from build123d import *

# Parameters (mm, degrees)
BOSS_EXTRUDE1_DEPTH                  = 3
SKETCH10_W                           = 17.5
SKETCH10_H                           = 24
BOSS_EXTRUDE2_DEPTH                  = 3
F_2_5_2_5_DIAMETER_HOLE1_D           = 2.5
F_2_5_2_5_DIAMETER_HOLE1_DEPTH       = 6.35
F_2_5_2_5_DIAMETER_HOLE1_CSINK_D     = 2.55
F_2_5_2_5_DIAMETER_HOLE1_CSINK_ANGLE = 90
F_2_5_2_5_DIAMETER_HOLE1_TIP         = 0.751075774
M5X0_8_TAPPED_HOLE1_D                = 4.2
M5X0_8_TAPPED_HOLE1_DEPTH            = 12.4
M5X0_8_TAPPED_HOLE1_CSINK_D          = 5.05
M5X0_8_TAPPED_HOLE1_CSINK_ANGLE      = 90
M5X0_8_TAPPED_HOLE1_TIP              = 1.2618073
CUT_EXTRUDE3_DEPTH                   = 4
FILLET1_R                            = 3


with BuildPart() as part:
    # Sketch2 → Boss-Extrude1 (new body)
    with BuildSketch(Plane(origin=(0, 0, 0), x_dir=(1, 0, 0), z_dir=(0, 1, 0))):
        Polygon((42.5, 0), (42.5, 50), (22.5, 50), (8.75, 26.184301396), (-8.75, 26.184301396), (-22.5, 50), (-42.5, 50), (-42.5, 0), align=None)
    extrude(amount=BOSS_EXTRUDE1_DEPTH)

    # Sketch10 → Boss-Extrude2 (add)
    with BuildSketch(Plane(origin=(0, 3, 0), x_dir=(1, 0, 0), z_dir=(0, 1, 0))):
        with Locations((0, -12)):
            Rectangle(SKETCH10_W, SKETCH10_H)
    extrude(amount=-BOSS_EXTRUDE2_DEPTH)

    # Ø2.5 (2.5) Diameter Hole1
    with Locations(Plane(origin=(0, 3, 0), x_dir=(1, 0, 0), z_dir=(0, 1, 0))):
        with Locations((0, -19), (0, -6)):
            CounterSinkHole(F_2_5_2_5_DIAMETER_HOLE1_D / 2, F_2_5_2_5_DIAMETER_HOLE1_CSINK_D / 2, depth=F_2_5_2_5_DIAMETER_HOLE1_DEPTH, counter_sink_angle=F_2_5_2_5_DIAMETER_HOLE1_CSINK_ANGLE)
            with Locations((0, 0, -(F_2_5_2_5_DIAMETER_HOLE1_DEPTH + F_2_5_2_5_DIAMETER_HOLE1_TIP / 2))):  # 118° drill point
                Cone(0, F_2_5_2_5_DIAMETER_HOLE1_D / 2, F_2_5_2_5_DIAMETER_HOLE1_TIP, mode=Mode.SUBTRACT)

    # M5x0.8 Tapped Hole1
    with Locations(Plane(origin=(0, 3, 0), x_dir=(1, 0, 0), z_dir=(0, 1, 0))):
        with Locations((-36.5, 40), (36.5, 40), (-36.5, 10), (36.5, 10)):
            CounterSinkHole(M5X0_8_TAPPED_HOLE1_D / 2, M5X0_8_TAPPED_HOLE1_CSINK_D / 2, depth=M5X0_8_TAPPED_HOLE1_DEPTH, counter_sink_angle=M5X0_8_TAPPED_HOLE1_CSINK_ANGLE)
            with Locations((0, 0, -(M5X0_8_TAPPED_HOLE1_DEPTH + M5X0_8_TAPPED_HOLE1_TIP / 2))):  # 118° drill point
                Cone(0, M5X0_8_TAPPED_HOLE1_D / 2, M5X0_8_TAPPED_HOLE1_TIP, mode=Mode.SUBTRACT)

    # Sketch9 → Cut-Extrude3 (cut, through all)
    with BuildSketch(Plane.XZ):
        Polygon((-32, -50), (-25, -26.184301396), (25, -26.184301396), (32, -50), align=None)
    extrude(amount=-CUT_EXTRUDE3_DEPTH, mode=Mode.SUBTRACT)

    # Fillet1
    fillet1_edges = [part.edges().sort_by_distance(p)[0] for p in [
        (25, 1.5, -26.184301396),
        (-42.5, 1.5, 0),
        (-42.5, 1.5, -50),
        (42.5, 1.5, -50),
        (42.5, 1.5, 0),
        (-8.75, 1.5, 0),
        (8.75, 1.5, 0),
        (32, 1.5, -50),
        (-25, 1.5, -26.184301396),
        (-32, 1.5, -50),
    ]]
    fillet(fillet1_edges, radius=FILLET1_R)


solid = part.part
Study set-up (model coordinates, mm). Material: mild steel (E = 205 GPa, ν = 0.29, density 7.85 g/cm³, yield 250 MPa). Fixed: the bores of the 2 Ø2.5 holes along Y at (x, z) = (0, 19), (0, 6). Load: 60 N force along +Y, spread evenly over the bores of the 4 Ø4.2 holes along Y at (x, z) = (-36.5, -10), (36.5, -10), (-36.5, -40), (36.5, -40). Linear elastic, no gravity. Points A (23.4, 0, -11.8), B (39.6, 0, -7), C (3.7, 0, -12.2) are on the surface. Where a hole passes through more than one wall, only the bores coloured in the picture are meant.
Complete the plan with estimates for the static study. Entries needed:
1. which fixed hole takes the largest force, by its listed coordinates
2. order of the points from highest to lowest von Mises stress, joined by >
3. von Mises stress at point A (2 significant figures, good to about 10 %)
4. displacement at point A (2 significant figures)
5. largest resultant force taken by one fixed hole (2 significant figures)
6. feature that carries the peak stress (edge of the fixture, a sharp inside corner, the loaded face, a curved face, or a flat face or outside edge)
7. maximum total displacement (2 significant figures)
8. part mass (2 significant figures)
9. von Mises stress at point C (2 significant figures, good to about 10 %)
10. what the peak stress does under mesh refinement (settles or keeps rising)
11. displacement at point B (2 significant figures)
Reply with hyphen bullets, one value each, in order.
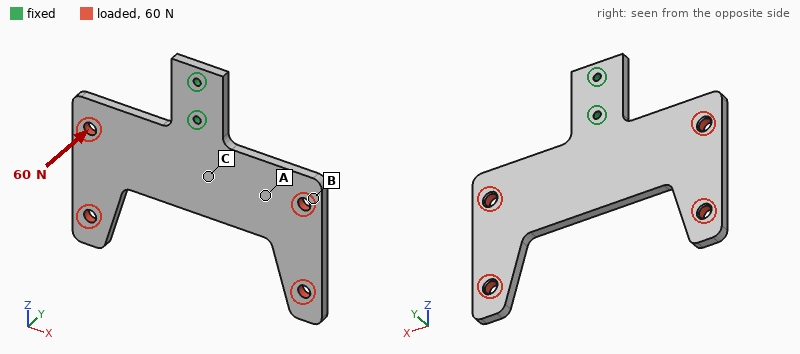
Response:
- (0, 6)
- C > A > B
- 10 MPa
- 0.041 mm
- 120 N
- edge of the fixture
- 0.17 mm
- 76 g
- 20 MPa
- keeps rising
- 0.050 mm
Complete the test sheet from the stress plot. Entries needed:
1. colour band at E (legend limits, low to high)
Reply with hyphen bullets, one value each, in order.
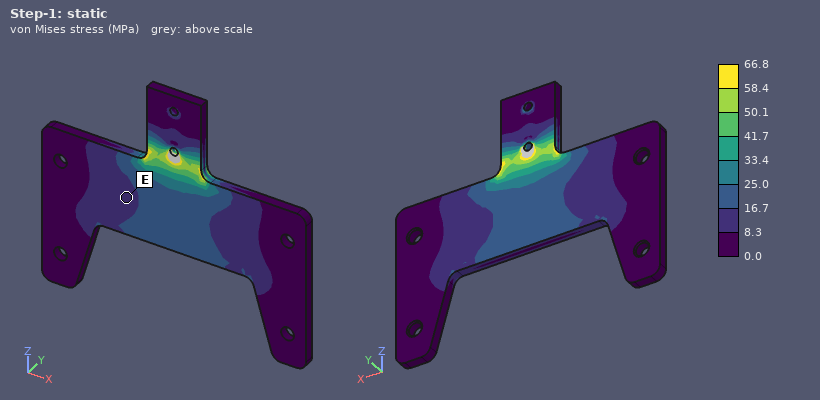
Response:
- 8.3 to 16.7 MPa
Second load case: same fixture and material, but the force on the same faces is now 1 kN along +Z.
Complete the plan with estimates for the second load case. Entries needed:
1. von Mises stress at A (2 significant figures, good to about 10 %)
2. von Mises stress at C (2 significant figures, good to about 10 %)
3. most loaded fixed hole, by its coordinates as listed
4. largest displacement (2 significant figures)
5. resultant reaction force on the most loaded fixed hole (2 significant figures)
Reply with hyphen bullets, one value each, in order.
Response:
- 19 MPa
- 7.8 MPa
- (0, 6)
- 30 µm
- 780 N
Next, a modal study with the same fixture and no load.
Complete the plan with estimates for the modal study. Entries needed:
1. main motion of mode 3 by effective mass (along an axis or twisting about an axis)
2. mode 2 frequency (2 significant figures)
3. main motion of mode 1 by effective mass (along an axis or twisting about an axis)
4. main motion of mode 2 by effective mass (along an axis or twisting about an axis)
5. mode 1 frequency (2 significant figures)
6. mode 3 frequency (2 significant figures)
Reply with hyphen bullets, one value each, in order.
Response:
- along X
- 620 Hz
- twisting about Z
- along Y
- 570 Hz
- 1900 Hz
